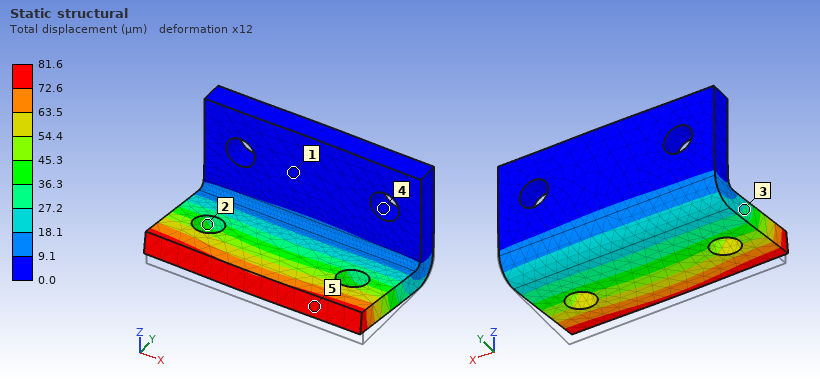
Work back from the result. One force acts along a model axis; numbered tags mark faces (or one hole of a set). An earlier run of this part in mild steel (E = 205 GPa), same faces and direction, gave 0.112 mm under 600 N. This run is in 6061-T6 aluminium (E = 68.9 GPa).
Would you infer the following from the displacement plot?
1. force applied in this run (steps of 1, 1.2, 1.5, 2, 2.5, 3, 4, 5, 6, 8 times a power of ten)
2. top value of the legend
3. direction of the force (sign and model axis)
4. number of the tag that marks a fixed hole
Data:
150 N
81.6 µm
+Z
4
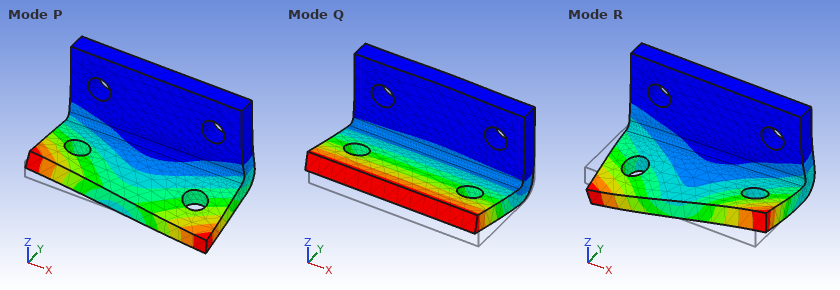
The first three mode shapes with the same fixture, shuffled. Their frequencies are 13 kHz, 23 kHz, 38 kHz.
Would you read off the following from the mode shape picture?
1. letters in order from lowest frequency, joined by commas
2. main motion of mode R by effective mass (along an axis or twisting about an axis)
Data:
Q, P, R
along X
